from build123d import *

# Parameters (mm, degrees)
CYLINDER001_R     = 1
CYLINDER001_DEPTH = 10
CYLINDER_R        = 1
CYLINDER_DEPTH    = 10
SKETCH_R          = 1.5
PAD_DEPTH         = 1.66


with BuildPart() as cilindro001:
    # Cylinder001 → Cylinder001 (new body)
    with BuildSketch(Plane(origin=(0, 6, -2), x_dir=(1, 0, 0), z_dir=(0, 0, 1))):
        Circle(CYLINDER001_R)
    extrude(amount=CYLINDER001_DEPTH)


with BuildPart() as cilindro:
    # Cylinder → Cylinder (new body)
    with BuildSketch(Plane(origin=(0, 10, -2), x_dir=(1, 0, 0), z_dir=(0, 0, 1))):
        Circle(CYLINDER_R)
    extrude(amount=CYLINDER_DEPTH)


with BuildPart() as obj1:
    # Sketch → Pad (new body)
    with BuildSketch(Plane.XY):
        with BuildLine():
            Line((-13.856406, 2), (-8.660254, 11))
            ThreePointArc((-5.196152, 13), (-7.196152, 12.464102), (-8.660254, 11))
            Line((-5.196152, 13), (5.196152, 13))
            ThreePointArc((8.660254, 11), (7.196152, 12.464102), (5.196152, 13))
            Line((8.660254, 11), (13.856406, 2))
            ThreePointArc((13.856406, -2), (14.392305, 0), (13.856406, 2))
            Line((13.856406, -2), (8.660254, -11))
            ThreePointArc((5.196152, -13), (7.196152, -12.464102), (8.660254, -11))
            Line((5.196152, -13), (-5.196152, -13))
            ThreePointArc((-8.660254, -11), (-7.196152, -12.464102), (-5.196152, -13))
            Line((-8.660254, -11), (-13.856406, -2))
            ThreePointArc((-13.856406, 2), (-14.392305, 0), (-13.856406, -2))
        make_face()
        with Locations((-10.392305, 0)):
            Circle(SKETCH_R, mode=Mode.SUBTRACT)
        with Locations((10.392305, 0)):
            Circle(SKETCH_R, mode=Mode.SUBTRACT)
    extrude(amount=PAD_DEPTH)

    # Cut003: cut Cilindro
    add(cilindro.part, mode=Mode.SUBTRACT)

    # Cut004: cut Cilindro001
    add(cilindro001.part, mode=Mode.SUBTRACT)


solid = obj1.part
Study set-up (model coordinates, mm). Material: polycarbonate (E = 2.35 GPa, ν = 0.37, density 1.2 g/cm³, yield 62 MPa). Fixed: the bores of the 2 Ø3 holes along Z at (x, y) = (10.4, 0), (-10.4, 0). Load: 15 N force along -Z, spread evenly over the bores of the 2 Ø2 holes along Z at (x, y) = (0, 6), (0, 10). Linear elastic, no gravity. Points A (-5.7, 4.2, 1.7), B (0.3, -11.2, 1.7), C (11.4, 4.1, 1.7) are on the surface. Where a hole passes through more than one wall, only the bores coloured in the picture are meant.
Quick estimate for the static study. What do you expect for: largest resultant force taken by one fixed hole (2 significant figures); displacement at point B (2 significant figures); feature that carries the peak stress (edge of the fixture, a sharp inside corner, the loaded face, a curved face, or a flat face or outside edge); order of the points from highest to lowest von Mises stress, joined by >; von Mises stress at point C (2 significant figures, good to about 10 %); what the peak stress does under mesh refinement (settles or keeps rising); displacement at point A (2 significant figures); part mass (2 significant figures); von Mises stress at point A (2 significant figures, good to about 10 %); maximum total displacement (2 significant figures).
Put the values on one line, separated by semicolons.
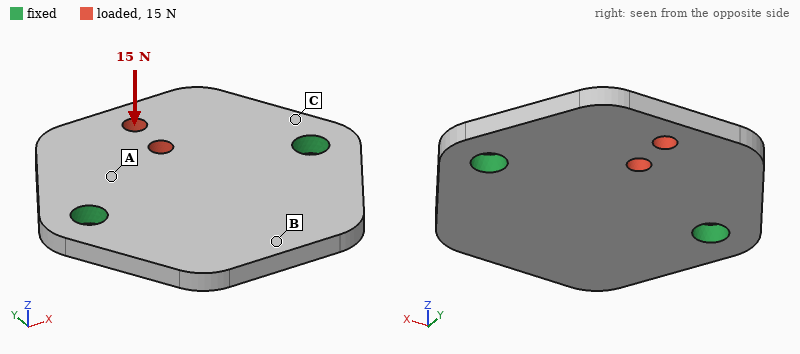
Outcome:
7.5 N; 0.065 mm; edge of the fixture; C > A > B; 9.2 MPa; keeps rising; 0.082 mm; 1.1 g; 5.1 MPa; 0.38 mm
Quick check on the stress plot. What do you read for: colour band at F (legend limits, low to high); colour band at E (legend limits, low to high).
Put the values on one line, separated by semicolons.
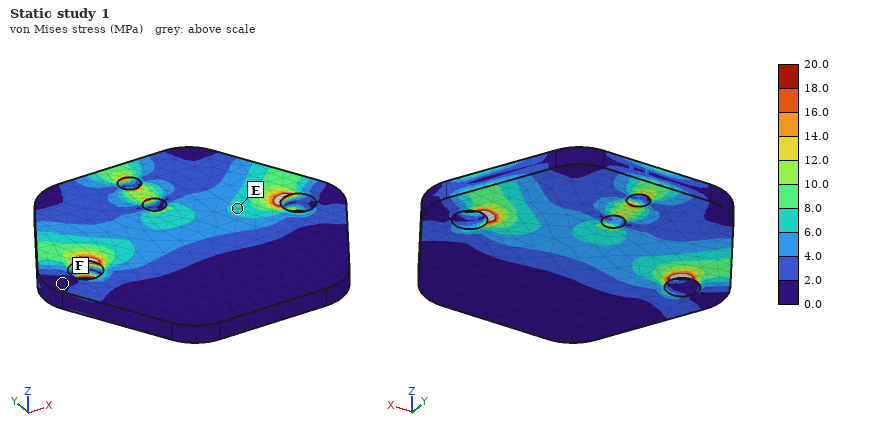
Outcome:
0.0 to 2.0 MPa; 6.0 to 8.0 MPa
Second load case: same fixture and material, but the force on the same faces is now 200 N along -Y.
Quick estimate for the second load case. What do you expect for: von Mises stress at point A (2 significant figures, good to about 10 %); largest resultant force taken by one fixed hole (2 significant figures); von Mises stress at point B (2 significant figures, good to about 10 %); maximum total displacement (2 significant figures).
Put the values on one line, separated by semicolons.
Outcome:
7.7 MPa; 100 N; 2.4 MPa; 69 µm
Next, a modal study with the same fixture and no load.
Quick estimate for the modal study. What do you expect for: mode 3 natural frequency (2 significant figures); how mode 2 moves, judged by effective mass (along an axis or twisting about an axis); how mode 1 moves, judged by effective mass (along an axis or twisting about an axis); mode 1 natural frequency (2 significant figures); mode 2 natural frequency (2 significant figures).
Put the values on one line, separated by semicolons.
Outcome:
5400 Hz; along Z; twisting about X; 2100 Hz; 2600 Hz
